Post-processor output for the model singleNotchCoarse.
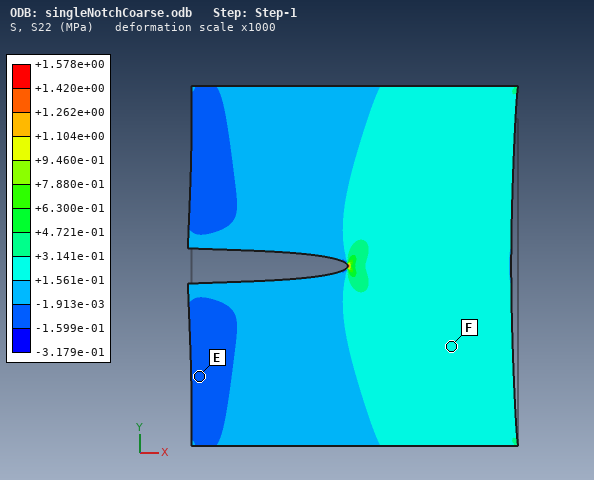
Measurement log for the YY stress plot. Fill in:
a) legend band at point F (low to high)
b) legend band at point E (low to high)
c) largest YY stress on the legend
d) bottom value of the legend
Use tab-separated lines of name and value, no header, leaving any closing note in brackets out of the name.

legend band at point F	+1.561e-01 to +3.141e-01 MPa
legend band at point E	-1.599e-01 to -1.913e-03 MPa
largest YY stress on the legend	+1.578e+00 MPa
bottom value of the legend	-3.179e-01 MPa
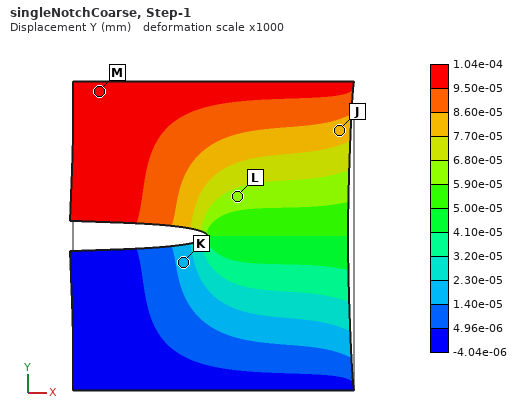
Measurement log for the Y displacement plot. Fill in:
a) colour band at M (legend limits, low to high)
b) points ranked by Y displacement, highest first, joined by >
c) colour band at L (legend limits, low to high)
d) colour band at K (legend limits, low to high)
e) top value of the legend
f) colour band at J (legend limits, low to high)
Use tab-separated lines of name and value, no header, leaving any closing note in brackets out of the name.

colour band at M	9.50e-05 to 1.04e-04 mm
points ranked by Y displacement, highest first, joined by >	M > J > L > K
colour band at L	5.90e-05 to 6.80e-05 mm
colour band at K	1.40e-05 to 2.30e-05 mm
top value of the legend	1.04e-04 mm
colour band at J	7.70e-05 to 8.60e-05 mm
